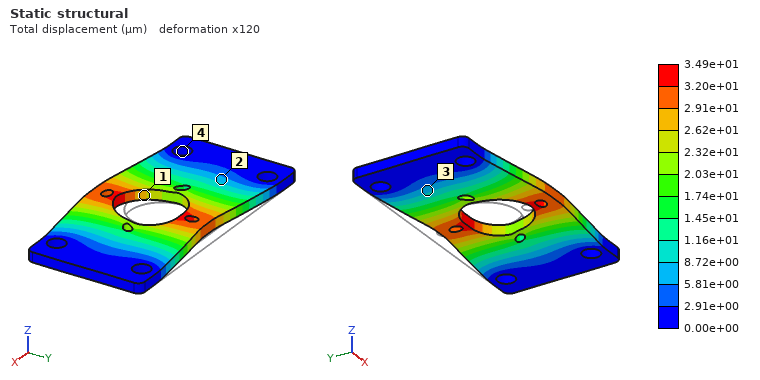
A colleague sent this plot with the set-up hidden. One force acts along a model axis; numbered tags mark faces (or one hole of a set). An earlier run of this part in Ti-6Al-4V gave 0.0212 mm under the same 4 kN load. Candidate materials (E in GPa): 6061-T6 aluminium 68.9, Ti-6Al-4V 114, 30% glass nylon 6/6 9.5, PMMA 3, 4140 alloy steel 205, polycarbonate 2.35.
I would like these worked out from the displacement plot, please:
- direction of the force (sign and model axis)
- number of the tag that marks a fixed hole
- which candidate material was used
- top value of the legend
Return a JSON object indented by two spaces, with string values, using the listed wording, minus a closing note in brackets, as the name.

{
  "direction of the force": "-Y",
  "number of the tag that marks a fixed hole": "4",
  "which candidate material was used": "6061-T6 aluminium",
  "top value of the legend": "3.49e+01 µm"
}
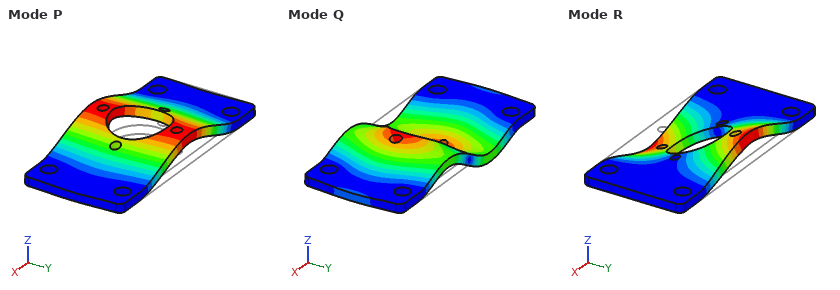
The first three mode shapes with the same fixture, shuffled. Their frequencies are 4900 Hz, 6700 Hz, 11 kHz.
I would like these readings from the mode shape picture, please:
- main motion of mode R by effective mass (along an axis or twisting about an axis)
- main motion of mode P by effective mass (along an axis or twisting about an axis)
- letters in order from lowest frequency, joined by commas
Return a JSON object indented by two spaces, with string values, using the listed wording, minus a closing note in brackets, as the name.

{
  "main motion of mode R by effective mass": "twisting about X",
  "main motion of mode P by effective mass": "along Z",
  "letters in order from lowest frequency, joined by commas": "P, R, Q"
}
